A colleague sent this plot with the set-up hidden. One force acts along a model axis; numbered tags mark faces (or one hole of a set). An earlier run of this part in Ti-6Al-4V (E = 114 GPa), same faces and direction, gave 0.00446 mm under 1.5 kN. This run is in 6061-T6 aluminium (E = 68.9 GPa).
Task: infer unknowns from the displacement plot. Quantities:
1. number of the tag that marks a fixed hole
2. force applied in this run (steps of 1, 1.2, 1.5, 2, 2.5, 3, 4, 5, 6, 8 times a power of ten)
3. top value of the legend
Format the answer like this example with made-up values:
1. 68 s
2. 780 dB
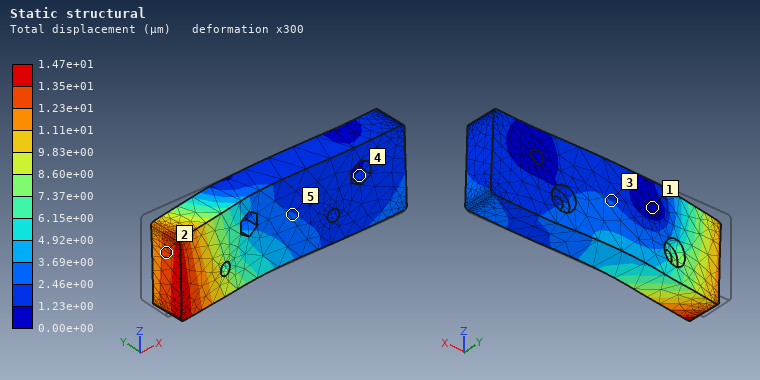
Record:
1. 1
2. 3 kN
3. 1.47e+01 µm
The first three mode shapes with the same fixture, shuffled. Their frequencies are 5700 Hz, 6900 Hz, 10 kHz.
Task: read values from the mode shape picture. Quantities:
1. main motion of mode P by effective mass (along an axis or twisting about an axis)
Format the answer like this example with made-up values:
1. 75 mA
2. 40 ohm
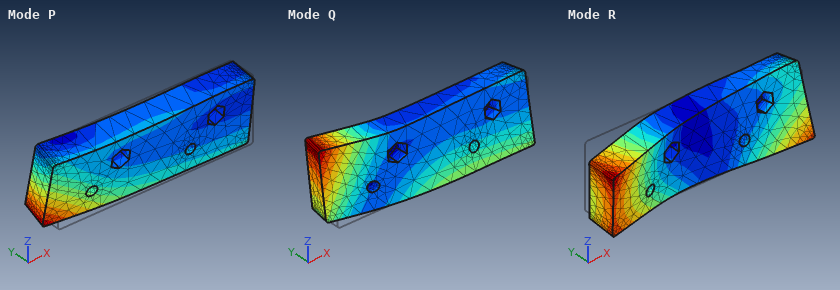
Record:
1. along Y
